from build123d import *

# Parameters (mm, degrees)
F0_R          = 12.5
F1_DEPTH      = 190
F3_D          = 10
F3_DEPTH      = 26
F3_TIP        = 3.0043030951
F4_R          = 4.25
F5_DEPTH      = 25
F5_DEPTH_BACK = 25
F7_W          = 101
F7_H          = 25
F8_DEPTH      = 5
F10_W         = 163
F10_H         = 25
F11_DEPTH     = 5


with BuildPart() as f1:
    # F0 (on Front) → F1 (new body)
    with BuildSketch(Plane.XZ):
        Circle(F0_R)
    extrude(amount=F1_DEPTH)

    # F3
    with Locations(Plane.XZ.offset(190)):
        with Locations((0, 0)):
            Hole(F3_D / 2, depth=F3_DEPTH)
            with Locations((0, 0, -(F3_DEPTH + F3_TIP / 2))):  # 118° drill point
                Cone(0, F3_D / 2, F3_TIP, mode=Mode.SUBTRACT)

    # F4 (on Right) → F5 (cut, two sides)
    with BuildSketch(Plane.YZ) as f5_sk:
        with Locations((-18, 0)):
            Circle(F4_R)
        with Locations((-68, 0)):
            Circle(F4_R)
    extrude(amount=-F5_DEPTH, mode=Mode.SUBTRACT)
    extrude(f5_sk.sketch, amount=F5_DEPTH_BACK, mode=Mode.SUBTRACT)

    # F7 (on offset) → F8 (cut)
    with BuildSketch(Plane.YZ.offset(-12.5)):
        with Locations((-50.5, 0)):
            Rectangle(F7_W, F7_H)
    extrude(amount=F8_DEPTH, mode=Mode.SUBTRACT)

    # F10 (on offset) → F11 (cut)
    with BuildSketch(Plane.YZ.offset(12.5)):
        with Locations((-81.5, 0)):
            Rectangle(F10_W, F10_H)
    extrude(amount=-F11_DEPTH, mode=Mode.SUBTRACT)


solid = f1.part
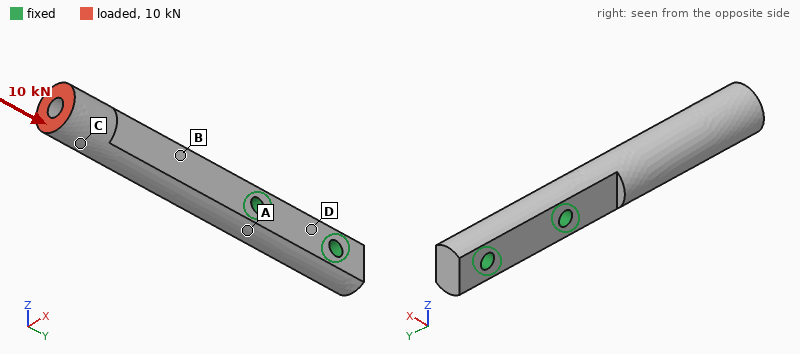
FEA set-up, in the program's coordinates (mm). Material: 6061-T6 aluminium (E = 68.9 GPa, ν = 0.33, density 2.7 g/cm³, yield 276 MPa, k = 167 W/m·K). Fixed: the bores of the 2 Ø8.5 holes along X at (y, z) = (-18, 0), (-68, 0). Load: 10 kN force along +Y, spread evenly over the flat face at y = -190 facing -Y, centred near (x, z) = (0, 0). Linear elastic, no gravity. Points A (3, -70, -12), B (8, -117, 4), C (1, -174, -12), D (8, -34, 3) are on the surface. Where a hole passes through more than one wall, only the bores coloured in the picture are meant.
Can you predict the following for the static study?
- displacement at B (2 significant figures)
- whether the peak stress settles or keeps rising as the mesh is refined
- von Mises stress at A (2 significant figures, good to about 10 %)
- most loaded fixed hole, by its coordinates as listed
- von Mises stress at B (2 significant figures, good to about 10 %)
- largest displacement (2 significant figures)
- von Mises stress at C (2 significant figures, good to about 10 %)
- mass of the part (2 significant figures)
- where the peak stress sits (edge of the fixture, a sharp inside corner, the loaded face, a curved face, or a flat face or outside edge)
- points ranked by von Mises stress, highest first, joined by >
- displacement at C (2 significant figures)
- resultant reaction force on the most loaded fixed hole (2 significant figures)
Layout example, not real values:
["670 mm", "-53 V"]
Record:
["22 µm", "keeps rising", "15 MPa", "(-68, 0)", "36 MPa", "95 µm", "27 MPa", "190 g", "edge of the fixture", "B > C > A > D", "65 µm", "9.6 kN"]
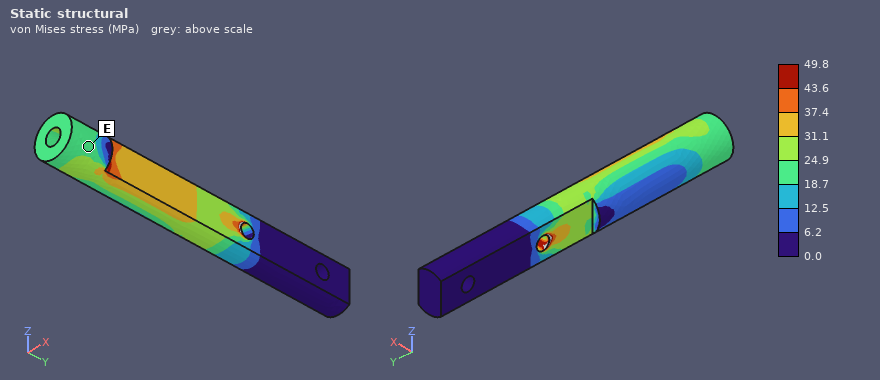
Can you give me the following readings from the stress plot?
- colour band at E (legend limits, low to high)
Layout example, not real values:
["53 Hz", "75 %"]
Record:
["18.7 to 24.9 MPa"]
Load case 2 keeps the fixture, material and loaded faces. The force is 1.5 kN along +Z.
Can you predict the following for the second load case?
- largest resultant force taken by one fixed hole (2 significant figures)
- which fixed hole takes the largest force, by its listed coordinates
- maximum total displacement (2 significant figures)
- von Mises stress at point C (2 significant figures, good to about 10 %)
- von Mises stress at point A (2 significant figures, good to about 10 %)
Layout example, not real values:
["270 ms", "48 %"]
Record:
["3.0 kN", "(-68, 0)", "0.94 mm", "16 MPa", "100 MPa"]
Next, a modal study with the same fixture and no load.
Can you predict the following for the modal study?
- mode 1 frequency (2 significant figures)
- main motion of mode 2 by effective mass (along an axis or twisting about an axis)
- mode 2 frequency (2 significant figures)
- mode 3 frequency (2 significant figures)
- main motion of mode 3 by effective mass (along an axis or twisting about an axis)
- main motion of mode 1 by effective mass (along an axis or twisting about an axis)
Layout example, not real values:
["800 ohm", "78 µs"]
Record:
["790 Hz", "along Z", "1100 Hz", "5100 Hz", "twisting about Y", "along X"]
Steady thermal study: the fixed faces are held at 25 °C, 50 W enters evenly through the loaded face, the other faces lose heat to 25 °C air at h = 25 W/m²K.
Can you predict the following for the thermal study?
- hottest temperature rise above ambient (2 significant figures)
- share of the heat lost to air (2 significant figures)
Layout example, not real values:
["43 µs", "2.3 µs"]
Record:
["78 K", "21 %"]
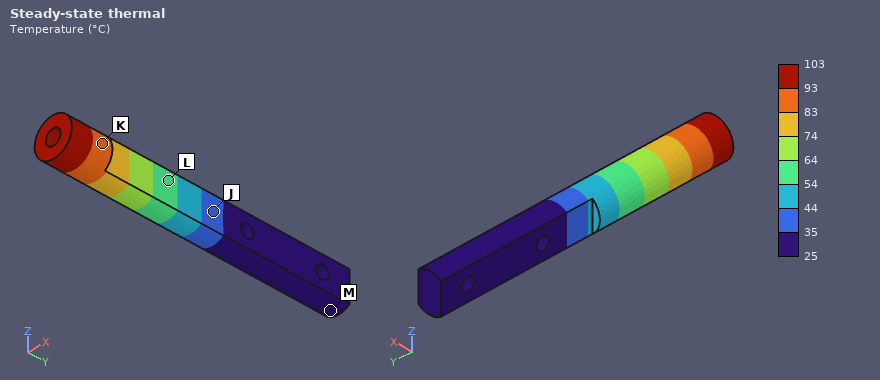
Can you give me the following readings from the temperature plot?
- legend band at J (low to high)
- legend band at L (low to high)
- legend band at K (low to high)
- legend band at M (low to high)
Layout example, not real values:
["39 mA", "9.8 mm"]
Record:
["35 to 44 °C", "54 to 64 °C", "83 to 93 °C", "25 to 35 °C"]
